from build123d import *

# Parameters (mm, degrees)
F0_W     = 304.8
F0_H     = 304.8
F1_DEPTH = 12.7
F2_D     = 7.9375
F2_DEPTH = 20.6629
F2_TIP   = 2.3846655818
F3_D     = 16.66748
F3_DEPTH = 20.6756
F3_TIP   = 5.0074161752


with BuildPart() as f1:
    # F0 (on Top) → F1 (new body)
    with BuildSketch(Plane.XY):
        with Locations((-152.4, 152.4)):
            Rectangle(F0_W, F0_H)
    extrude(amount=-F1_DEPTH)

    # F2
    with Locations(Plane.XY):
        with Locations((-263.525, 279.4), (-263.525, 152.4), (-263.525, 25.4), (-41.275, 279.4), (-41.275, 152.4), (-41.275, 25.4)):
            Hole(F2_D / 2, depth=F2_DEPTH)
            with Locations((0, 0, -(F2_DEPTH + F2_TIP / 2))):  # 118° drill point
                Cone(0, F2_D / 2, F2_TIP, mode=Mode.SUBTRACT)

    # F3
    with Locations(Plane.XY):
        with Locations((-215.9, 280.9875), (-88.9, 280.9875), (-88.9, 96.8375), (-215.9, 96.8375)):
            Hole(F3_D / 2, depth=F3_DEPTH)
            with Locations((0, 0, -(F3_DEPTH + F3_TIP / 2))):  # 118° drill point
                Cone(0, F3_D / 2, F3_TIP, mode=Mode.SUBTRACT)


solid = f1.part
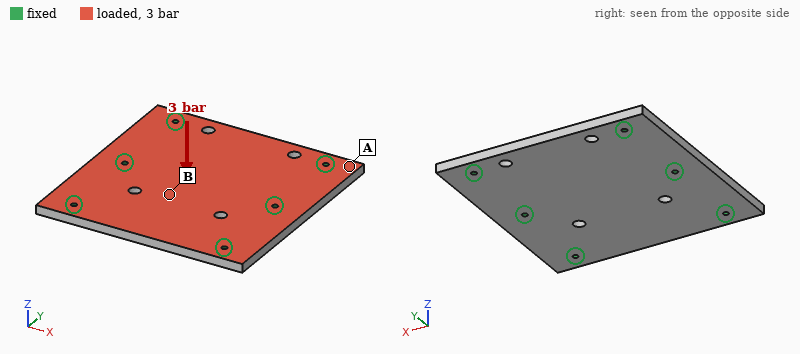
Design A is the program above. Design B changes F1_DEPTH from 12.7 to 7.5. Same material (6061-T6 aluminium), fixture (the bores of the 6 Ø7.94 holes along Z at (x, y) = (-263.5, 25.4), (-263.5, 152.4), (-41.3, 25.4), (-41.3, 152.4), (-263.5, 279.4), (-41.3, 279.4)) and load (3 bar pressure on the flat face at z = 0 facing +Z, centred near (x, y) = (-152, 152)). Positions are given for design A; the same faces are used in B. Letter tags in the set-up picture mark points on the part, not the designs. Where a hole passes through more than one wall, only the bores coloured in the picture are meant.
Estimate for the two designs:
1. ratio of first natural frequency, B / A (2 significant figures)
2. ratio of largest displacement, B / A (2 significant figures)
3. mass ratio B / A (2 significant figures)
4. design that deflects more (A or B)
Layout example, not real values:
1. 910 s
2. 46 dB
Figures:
1. 0.63
2. 4.4
3. 0.59
4. B
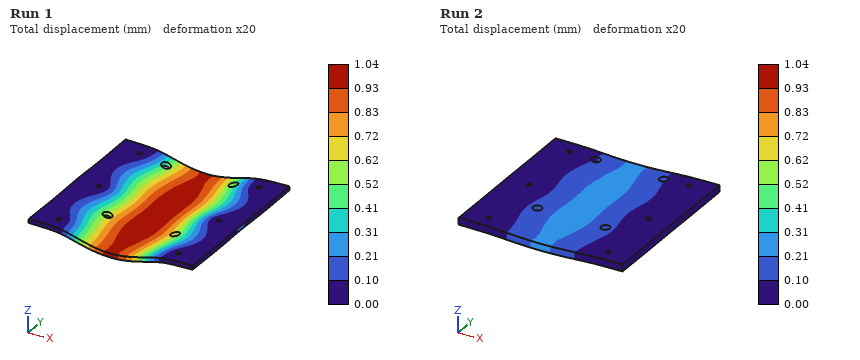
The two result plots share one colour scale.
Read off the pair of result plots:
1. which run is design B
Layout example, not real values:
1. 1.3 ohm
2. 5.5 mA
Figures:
1. Run 1
